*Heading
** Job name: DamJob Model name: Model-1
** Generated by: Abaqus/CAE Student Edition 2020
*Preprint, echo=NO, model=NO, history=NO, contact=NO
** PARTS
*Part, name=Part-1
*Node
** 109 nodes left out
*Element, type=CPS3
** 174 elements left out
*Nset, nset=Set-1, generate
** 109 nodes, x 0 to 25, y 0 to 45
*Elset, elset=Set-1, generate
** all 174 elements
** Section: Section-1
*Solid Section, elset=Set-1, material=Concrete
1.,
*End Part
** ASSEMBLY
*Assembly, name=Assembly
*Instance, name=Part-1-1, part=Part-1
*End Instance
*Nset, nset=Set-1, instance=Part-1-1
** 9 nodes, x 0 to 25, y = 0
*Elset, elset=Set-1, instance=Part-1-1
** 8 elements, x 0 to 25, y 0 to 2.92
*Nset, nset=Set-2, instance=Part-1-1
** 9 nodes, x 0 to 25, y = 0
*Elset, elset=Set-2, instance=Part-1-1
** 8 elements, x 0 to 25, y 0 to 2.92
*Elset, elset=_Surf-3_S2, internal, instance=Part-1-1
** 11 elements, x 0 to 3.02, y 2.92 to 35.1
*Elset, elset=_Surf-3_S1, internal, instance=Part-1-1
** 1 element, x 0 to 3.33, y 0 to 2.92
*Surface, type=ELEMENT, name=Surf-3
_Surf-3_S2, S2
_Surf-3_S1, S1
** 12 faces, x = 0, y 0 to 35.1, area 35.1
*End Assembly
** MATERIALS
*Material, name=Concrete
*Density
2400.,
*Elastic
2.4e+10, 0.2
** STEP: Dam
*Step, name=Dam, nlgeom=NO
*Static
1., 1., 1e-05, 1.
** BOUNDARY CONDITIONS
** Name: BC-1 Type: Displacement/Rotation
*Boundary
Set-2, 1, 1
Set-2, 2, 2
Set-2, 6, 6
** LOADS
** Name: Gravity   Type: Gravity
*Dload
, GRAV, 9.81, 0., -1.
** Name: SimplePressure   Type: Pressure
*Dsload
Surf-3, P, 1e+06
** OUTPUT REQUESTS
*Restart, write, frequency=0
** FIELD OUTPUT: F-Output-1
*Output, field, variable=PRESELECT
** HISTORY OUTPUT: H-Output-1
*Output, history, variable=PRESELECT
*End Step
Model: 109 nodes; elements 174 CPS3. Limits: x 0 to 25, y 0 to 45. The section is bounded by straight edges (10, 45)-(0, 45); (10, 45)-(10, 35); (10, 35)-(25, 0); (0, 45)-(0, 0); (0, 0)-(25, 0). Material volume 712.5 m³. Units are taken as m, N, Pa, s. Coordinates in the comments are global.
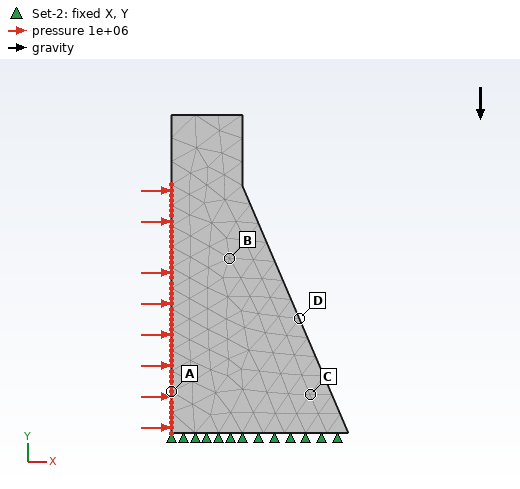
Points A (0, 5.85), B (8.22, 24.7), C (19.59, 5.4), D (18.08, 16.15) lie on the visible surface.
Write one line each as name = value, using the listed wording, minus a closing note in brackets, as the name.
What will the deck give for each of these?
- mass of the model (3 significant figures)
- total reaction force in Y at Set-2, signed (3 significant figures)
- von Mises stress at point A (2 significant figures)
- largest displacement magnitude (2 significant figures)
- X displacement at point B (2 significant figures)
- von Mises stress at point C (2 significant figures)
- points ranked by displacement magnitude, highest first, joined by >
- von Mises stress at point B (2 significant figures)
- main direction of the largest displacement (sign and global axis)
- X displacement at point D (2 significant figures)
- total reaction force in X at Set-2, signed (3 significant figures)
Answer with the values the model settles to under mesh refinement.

mass of the model = 1.71e+06 kg
total reaction force in Y at Set-2, signed = 1.68e+07 N
von Mises stress at point A = 4.7e+06 Pa
largest displacement magnitude = 0.017 m
X displacement at point B = 0.0081 m
von Mises stress at point C = 4.5e+06 Pa
points ranked by displacement magnitude, highest first, joined by > = B > D > A > C
von Mises stress at point B = 1.7e+06 Pa
main direction of the largest displacement = +X
X displacement at point D = 0.0042 m
total reaction force in X at Set-2, signed = -3.51e+07 N
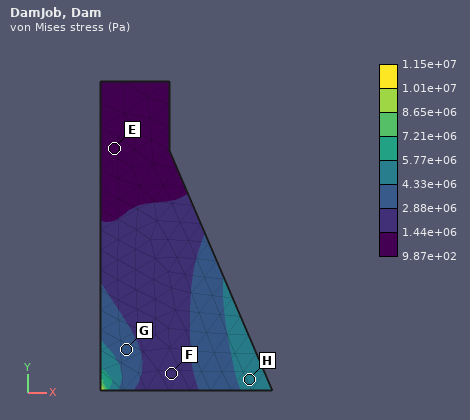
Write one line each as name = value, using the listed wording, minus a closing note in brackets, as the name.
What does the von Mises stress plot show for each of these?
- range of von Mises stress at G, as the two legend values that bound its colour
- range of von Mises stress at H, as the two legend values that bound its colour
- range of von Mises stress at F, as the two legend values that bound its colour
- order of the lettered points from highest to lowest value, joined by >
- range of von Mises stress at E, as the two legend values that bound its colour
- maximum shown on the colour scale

range of von Mises stress at G, as the two legend values that bound its colour = 2.88e+06 to 4.33e+06 Pa
range of von Mises stress at H, as the two legend values that bound its colour = 4.33e+06 to 5.77e+06 Pa
range of von Mises stress at F, as the two legend values that bound its colour = 1.44e+06 to 2.88e+06 Pa
order of the lettered points from highest to lowest value, joined by > = H > G > F > E
range of von Mises stress at E, as the two legend values that bound its colour = 9.87e+02 to 1.44e+06 Pa
maximum shown on the colour scale = 1.15e+07 Pa
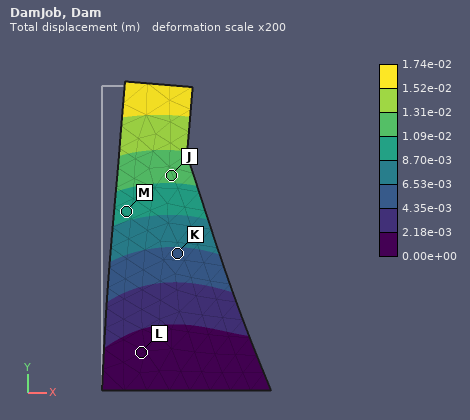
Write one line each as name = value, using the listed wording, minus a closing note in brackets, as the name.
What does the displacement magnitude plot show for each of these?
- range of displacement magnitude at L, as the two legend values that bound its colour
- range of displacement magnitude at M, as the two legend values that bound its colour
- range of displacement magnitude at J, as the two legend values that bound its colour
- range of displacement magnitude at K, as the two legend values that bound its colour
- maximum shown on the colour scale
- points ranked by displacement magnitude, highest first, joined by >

range of displacement magnitude at L, as the two legend values that bound its colour = 0.00e+00 to 2.18e-03 m
range of displacement magnitude at M, as the two legend values that bound its colour = 8.70e-03 to 1.09e-02 m
range of displacement magnitude at J, as the two legend values that bound its colour = 1.09e-02 to 1.31e-02 m
range of displacement magnitude at K, as the two legend values that bound its colour = 4.35e-03 to 6.53e-03 m
maximum shown on the colour scale = 1.74e-02 m
points ranked by displacement magnitude, highest first, joined by > = J > M > K > L
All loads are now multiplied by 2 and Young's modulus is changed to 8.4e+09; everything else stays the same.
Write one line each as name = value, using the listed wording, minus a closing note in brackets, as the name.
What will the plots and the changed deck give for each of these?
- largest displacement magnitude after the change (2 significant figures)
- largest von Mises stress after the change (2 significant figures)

largest displacement magnitude after the change = 0.099 m
largest von Mises stress after the change = 2.3e+07 Pa
